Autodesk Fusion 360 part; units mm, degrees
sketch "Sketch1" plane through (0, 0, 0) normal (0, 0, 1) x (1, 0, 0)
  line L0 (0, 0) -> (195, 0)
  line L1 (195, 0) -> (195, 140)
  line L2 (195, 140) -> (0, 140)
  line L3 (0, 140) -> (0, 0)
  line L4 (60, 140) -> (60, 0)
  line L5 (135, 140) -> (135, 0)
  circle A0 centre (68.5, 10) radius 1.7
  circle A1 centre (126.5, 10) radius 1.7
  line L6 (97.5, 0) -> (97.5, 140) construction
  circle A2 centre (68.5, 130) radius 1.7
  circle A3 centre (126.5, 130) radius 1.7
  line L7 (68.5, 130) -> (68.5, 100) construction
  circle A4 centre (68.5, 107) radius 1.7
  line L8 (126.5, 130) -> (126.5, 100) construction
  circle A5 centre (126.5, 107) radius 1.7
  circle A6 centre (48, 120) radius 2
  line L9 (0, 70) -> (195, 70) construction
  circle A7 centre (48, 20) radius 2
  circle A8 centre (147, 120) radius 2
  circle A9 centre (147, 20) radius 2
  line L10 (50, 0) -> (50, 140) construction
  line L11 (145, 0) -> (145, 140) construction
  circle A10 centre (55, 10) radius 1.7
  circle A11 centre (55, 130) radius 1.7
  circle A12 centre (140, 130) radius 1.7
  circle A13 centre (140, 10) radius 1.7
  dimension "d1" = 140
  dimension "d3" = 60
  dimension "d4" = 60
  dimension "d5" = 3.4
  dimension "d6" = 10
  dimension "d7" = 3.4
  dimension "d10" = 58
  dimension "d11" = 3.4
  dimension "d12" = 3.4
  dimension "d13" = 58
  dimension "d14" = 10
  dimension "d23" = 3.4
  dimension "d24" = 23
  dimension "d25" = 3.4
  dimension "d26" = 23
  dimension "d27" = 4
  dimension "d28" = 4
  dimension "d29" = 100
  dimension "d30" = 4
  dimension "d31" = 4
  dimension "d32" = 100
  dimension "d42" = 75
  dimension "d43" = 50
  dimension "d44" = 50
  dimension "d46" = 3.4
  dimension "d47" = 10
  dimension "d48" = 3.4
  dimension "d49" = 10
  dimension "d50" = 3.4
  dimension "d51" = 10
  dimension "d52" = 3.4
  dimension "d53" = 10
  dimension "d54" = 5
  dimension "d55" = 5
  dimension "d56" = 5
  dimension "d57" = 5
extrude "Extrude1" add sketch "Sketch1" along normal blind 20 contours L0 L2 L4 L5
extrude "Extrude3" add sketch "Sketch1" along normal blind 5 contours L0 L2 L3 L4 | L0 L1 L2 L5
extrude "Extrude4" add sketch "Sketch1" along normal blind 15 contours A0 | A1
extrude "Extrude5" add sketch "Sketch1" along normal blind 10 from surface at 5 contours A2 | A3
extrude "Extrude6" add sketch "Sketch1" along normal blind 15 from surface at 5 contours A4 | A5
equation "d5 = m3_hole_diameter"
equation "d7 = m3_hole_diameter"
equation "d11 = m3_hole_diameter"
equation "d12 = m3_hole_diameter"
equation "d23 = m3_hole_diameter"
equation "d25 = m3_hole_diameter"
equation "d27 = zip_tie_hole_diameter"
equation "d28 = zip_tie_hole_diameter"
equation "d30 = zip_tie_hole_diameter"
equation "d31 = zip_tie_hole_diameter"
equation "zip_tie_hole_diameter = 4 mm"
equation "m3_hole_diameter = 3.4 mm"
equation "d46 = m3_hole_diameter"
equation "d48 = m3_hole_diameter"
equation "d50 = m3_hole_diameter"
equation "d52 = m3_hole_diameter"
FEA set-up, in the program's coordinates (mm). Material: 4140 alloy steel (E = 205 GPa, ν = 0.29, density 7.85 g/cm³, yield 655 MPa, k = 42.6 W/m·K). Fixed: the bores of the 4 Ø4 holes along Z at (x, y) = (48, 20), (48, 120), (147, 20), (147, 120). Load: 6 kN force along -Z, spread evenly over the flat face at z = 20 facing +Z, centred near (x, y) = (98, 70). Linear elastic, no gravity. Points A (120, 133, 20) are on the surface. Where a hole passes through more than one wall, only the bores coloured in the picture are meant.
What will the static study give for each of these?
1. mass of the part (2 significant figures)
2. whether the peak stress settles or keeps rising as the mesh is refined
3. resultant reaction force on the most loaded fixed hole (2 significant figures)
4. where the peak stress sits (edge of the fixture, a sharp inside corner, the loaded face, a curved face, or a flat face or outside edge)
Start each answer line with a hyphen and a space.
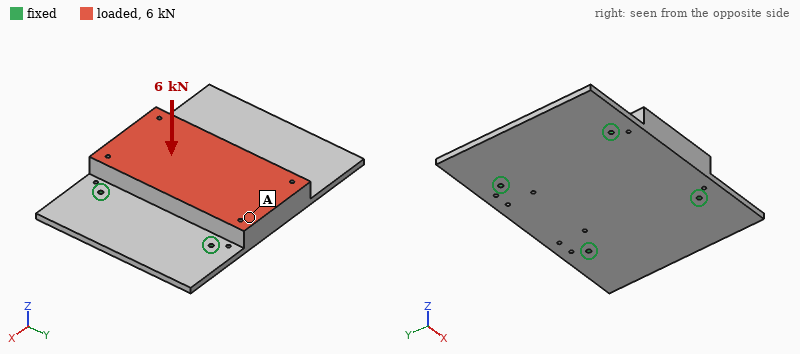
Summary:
- 2.3 kg
- keeps rising
- 1.9 kN
- edge of the fixture
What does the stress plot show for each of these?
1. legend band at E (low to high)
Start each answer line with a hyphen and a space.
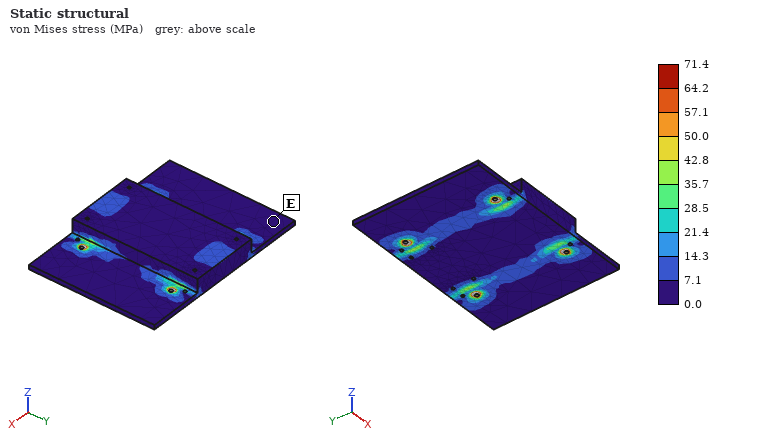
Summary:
- 0.0 to 7.1 MPa
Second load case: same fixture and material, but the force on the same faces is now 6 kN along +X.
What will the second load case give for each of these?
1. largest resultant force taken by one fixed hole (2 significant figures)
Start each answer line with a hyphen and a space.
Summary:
- 1.6 kN
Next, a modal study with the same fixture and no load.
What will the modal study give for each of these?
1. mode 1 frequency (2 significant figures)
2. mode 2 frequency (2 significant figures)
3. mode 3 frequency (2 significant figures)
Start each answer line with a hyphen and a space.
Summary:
- 1400 Hz
- 1400 Hz
- 2100 Hz
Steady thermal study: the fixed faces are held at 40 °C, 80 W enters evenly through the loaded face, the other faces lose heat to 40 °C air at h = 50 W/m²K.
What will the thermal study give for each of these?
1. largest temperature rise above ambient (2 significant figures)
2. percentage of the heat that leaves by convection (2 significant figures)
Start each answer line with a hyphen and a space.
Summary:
- 33 K
- 55 %
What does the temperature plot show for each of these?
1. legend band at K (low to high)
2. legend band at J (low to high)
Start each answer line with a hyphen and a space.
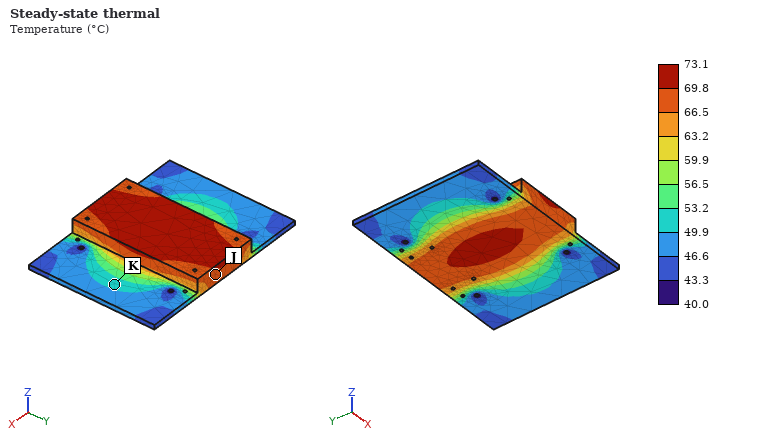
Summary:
- 49.9 to 53.2 °C
- 66.5 to 69.8 °C
